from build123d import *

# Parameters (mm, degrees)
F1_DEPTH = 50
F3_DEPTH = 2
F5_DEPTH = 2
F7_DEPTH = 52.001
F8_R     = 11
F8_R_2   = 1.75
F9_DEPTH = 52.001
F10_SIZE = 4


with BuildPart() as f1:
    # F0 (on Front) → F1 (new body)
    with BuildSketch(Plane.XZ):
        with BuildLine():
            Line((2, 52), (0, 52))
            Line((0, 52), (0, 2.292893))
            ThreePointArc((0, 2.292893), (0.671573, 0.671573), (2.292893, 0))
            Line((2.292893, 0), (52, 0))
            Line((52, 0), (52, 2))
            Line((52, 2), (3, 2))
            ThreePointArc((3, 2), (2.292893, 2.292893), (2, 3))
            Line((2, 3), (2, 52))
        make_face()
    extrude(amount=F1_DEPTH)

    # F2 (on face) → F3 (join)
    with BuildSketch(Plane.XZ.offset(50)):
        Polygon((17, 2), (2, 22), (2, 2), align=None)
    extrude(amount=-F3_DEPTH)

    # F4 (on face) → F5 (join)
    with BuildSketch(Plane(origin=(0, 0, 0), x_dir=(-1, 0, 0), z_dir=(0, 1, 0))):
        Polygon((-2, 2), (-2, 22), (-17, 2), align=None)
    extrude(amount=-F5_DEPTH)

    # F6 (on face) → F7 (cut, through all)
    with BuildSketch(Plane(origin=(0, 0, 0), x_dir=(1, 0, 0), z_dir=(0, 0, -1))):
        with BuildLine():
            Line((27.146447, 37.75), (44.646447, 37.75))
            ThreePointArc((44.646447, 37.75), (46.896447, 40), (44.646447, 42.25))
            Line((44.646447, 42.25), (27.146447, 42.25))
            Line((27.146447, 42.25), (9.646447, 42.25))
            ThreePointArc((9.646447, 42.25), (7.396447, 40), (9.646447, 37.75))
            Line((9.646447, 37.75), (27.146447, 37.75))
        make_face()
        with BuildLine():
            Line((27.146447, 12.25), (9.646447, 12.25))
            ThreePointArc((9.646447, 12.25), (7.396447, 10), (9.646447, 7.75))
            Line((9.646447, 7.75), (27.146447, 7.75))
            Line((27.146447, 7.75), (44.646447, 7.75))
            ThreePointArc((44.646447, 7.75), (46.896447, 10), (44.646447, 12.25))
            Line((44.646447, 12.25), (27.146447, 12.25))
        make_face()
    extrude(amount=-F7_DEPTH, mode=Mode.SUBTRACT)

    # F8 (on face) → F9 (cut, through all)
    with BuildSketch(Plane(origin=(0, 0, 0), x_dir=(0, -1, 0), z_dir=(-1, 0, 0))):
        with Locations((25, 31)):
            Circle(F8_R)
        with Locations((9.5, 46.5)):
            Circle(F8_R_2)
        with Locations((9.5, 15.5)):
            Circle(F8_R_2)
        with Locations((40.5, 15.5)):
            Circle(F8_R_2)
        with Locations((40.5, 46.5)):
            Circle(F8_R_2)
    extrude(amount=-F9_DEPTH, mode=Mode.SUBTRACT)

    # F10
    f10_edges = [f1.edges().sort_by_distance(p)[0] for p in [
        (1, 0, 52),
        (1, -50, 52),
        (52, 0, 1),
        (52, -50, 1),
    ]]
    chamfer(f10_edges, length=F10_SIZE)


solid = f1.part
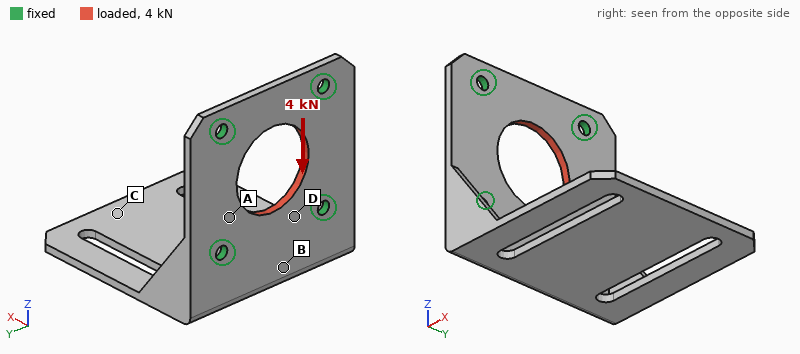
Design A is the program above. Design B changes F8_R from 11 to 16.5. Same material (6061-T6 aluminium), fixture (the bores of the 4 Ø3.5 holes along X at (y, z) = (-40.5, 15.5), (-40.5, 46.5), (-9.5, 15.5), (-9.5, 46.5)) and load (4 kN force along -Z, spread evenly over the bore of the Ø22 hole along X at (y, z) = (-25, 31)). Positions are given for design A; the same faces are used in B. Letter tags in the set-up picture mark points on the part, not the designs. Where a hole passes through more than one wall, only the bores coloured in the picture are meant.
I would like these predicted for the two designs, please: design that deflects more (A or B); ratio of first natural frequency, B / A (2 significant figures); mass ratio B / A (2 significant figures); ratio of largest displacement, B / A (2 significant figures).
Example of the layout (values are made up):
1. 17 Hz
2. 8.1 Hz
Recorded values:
1. B
2. 0.98
3. 0.90
4. 1.8
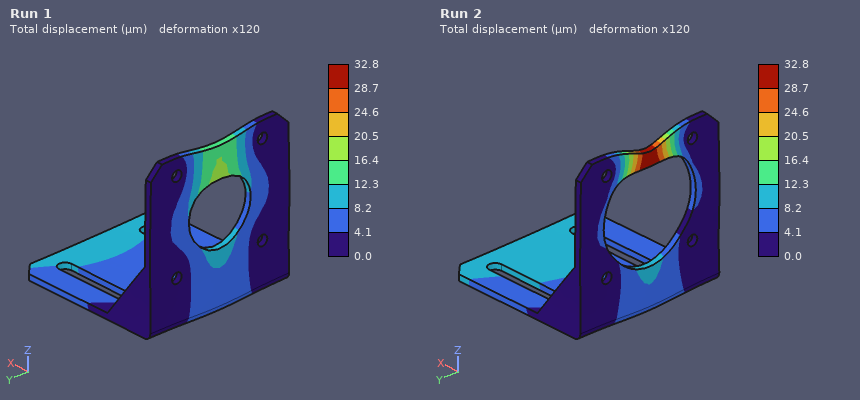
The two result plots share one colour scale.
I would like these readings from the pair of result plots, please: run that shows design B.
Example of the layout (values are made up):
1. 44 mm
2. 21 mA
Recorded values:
1. Run 2
